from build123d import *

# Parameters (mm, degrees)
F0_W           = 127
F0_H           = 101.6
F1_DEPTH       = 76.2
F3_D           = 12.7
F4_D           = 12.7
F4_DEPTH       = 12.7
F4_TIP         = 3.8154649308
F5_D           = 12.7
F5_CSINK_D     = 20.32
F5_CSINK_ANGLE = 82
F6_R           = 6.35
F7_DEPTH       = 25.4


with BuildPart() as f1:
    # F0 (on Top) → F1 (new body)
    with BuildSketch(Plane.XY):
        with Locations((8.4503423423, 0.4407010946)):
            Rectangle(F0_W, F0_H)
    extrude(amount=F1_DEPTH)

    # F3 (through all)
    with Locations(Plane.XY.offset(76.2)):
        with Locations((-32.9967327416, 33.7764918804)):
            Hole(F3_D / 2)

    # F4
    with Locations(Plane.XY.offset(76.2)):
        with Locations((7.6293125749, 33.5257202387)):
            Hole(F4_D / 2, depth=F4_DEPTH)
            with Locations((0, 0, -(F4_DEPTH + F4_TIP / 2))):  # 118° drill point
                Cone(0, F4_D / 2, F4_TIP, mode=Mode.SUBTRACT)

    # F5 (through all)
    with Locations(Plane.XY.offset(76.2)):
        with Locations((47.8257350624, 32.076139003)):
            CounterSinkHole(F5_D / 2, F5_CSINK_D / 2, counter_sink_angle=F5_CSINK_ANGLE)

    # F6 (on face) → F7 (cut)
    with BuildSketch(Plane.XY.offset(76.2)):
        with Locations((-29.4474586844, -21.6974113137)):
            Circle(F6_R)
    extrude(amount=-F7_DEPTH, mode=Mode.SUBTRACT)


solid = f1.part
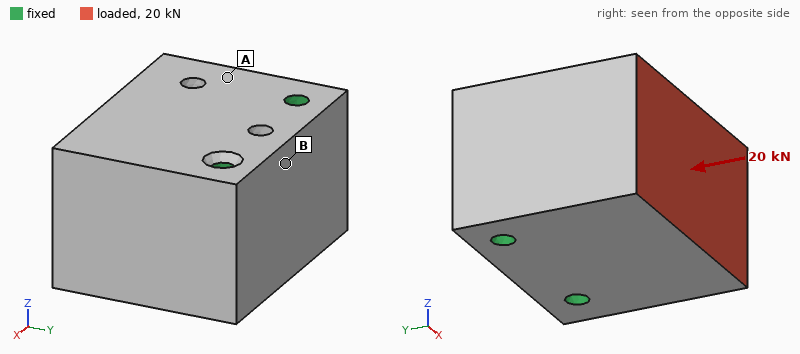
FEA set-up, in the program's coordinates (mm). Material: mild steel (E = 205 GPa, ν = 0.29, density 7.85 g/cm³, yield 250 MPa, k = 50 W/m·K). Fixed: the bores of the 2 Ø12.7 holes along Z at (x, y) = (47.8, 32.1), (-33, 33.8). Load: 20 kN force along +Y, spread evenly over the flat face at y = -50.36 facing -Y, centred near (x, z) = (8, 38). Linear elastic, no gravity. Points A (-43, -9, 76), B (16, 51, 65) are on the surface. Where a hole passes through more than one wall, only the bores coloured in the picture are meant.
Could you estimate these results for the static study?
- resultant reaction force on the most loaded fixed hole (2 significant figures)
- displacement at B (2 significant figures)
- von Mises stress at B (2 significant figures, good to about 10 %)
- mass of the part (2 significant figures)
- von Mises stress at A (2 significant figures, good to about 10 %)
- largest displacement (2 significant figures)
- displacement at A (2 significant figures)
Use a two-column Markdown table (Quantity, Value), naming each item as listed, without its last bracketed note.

| Quantity | Value |
|---|---|
| resultant reaction force on the most loaded fixed hole | 10 kN |
| displacement at B | 0.41 µm |
| von Mises stress at B | 1.3 MPa |
| mass of the part | 7.5 kg |
| von Mises stress at A | 2.6 MPa |
| largest displacement | 1.1 µm |
| displacement at A | 0.61 µm |
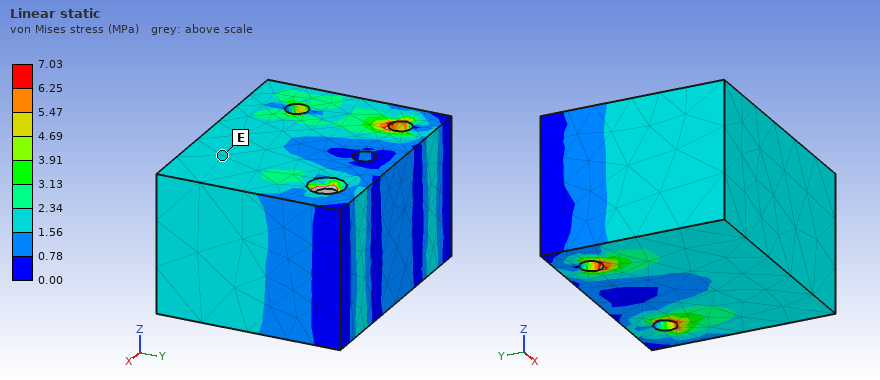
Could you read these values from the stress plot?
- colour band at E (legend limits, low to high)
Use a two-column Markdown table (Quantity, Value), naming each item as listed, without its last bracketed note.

| Quantity | Value |
|---|---|
| colour band at E | 1.56 to 2.34 MPa |
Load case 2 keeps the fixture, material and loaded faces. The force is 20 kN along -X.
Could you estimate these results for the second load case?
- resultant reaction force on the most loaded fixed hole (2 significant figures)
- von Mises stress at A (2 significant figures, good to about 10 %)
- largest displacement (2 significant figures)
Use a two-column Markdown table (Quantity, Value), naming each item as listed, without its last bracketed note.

| Quantity | Value |
|---|---|
| resultant reaction force on the most loaded fixed hole | 21 kN |
| von Mises stress at A | 3.0 MPa |
| largest displacement | 5.7 µm |
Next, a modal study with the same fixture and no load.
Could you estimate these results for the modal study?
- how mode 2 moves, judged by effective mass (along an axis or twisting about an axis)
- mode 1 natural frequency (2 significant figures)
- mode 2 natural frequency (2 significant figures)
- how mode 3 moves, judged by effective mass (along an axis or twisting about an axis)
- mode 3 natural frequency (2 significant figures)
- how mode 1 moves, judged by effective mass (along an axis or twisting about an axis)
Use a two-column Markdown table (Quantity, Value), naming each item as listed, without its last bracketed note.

| Quantity | Value |
|---|---|
| how mode 2 moves, judged by effective mass | along X |
| mode 1 natural frequency | 5200 Hz |
| mode 2 natural frequency | 6800 Hz |
| how mode 3 moves, judged by effective mass | twisting about Y |
| mode 3 natural frequency | 8200 Hz |
| how mode 1 moves, judged by effective mass | along Z |
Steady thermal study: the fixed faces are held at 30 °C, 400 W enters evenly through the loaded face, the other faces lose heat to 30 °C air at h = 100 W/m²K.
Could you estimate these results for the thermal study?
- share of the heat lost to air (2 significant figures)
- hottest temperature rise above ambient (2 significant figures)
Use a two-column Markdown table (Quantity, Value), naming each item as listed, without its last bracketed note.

| Quantity | Value |
|---|---|
| share of the heat lost to air | 28 % |
| hottest temperature rise above ambient | 62 K |
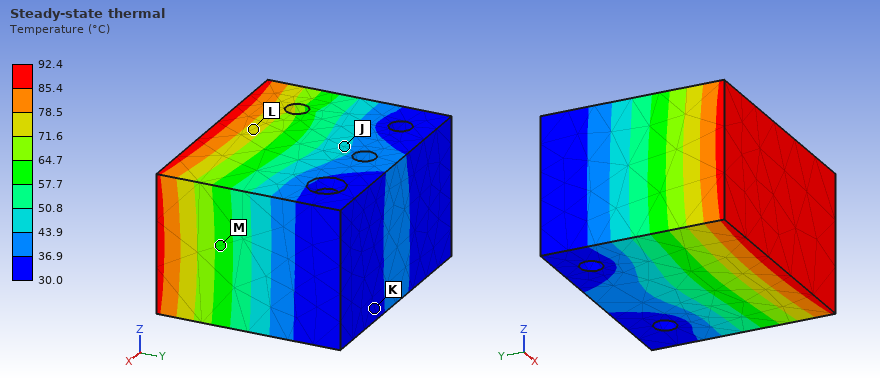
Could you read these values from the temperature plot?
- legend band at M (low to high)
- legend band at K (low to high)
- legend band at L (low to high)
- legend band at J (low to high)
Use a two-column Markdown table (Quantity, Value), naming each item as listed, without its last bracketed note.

| Quantity | Value |
|---|---|
| legend band at M | 57.7 to 64.7 °C |
| legend band at K | 30.0 to 36.9 °C |
| legend band at L | 71.6 to 78.5 °C |
| legend band at J | 43.9 to 50.8 °C |
